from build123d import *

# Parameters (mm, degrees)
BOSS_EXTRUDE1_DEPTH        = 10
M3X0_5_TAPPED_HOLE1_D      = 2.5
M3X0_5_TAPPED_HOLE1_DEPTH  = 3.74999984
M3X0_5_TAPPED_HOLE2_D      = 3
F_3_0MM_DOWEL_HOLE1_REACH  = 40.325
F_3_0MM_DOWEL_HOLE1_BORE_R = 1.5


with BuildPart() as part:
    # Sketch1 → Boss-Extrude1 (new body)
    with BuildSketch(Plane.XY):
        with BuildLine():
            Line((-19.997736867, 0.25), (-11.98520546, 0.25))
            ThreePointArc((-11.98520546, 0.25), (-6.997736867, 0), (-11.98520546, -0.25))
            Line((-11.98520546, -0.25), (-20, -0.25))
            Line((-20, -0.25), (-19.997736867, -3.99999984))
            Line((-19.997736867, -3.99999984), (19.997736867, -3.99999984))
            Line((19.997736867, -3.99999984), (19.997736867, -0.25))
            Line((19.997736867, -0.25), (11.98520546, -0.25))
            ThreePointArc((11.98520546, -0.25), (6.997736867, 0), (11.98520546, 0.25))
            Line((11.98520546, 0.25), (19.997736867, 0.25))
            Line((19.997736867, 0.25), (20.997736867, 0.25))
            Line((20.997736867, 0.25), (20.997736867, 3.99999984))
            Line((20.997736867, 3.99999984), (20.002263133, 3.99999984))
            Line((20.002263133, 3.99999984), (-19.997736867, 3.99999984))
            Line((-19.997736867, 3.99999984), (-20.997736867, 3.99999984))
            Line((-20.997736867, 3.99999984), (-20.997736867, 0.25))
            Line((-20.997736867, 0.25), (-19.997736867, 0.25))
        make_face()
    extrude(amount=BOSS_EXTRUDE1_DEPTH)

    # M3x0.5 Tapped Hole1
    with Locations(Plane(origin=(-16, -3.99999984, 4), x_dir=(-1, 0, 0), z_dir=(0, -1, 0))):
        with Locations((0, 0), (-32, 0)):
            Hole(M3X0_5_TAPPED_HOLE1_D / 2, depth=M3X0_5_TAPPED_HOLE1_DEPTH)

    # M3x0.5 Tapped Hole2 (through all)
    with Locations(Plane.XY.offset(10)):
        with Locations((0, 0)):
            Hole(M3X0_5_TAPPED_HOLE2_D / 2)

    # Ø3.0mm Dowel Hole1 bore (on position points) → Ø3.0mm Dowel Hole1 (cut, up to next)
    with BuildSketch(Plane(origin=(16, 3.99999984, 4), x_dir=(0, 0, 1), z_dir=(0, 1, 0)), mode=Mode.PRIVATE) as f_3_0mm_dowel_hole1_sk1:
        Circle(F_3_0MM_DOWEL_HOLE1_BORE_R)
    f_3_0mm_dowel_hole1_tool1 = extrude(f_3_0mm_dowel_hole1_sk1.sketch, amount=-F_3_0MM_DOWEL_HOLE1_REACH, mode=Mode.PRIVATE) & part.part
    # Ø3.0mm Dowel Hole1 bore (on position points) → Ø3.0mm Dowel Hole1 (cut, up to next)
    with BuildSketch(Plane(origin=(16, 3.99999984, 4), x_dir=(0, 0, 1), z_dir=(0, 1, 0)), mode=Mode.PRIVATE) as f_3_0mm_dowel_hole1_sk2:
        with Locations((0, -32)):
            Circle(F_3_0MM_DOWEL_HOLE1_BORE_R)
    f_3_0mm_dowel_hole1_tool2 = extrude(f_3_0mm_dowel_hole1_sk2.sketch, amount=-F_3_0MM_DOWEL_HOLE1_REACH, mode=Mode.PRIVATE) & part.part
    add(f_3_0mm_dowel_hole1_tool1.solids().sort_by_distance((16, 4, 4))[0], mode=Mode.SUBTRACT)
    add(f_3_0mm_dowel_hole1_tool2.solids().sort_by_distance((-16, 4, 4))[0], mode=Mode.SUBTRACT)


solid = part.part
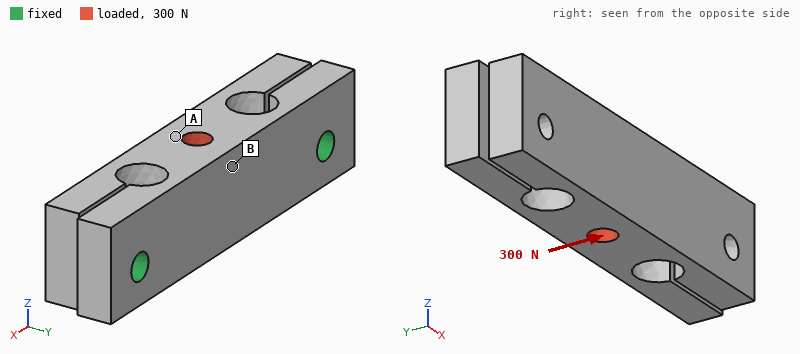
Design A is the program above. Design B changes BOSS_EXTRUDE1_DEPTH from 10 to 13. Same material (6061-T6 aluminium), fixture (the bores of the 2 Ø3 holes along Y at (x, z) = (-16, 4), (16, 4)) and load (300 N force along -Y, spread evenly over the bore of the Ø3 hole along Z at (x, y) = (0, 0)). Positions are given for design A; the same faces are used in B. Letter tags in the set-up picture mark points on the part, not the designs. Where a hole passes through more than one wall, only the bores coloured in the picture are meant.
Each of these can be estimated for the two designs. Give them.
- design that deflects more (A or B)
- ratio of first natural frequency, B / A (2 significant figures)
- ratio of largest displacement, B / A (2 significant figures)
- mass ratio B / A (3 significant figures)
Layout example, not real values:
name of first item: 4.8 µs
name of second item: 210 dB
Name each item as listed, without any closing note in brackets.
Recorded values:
design that deflects more: B
ratio of first natural frequency, B / A: 0.99
ratio of largest displacement, B / A: 1.1
mass ratio B / A: 1.31
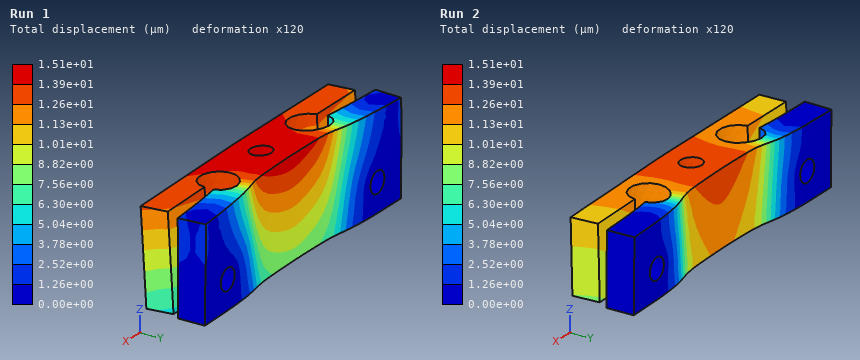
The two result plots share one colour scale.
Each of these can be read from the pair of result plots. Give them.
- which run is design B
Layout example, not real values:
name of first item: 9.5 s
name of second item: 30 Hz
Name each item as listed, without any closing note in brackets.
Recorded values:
which run is design B: Run 1
